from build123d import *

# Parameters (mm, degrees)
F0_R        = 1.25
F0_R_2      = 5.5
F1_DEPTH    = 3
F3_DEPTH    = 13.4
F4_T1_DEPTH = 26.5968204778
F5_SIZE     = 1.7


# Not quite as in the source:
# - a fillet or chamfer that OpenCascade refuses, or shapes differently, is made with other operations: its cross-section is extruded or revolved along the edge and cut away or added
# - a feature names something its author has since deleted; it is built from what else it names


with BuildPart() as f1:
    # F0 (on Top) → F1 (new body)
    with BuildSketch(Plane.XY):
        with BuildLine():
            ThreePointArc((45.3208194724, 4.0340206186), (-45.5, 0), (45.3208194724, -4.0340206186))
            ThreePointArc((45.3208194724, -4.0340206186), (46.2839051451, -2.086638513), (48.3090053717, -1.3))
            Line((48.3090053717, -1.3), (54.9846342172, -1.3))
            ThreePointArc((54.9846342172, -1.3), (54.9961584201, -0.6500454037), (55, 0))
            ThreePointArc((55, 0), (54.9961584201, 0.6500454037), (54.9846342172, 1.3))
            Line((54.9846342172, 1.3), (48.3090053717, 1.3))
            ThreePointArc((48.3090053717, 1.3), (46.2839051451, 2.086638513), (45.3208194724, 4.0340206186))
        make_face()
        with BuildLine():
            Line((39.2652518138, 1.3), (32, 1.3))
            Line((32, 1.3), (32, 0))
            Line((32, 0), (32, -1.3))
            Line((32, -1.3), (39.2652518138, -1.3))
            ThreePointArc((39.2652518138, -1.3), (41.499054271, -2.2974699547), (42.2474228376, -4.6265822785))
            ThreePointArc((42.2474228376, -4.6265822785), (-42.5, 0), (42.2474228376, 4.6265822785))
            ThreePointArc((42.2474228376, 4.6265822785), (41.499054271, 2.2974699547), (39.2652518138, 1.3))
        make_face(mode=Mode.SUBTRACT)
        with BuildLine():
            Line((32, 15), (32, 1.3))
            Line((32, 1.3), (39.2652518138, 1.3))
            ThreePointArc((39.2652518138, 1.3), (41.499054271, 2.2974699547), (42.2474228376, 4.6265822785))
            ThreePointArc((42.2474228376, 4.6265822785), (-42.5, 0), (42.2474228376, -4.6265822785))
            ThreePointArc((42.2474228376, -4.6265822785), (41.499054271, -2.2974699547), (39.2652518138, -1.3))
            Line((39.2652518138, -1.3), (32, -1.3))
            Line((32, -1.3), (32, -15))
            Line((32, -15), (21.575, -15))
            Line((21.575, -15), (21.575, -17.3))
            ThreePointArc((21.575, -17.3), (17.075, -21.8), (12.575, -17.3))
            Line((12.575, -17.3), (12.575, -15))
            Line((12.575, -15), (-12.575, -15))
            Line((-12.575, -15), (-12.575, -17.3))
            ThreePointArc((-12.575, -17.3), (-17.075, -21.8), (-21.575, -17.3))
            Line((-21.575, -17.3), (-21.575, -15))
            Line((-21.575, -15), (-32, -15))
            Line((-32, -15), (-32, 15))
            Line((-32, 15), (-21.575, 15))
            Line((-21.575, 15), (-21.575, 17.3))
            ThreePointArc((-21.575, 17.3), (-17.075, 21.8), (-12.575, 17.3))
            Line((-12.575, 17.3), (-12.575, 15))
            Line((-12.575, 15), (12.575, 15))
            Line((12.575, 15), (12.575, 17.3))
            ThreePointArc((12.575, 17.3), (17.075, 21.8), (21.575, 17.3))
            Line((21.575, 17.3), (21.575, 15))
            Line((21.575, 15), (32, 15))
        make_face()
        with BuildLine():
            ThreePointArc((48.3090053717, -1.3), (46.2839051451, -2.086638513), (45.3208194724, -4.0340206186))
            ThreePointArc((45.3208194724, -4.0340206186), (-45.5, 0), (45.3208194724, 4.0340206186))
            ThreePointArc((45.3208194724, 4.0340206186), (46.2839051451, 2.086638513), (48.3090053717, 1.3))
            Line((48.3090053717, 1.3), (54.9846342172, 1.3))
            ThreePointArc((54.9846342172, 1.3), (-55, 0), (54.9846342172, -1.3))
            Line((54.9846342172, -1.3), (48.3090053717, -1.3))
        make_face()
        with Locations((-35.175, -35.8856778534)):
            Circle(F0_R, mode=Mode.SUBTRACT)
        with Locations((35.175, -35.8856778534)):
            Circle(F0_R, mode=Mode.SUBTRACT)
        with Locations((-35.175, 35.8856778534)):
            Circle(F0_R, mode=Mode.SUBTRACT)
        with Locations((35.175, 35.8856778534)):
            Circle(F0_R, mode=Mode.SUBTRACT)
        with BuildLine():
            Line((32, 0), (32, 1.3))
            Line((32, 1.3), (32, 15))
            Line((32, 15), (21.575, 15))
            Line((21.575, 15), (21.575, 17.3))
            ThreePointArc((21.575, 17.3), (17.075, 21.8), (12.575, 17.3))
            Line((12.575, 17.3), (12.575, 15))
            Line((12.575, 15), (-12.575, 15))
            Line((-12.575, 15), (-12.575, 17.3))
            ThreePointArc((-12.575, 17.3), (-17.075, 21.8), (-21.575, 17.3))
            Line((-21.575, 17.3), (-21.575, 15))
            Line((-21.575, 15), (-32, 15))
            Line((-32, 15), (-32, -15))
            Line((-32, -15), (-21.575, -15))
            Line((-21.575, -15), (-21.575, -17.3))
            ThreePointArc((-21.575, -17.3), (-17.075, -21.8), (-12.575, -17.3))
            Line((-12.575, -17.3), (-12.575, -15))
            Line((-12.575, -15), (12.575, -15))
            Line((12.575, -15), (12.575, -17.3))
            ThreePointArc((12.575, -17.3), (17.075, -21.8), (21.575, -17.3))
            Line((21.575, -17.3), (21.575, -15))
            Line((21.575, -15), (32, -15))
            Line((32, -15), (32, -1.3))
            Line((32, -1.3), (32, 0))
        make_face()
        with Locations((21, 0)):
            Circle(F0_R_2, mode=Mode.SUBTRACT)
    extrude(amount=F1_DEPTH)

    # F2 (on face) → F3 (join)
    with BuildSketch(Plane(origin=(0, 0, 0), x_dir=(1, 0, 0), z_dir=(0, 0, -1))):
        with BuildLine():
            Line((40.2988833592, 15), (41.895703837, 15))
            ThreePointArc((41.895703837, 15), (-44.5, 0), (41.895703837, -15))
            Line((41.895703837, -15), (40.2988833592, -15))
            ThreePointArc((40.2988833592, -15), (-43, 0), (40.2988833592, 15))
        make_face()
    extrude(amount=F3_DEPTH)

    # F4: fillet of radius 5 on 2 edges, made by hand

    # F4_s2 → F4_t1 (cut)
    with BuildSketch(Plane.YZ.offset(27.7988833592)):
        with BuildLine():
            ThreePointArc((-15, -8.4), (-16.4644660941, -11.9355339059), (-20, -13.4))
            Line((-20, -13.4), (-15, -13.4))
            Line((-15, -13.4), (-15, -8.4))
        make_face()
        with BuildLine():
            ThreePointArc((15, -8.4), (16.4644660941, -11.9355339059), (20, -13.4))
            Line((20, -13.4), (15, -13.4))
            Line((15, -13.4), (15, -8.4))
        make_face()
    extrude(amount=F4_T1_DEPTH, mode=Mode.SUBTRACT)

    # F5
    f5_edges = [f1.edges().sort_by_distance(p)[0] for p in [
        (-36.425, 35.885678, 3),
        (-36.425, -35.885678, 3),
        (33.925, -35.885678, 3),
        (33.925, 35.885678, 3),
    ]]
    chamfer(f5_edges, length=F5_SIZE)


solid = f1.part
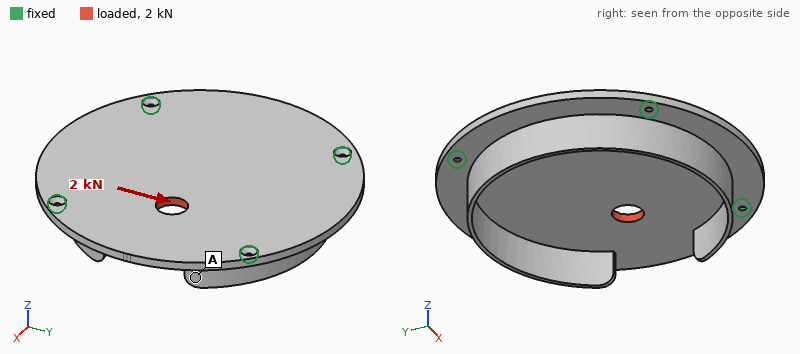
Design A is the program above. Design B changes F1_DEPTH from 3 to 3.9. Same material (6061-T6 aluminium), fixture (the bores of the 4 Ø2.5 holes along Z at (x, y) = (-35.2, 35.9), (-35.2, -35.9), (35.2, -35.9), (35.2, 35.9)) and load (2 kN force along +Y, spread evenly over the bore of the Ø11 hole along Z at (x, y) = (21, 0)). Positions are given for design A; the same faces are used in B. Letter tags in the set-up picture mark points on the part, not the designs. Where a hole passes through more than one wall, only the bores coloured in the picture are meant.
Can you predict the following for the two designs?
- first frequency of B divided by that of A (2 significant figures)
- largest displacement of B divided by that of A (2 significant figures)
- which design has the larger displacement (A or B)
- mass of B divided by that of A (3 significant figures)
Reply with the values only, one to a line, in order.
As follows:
1.3
0.73
A
1.26
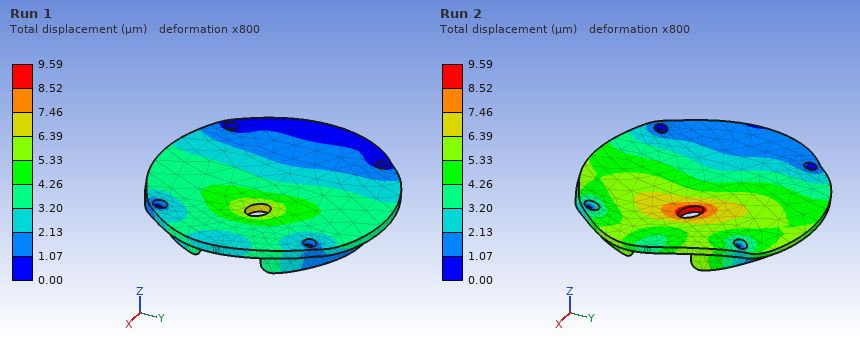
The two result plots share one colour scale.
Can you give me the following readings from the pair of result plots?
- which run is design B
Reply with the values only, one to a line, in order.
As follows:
Run 1
